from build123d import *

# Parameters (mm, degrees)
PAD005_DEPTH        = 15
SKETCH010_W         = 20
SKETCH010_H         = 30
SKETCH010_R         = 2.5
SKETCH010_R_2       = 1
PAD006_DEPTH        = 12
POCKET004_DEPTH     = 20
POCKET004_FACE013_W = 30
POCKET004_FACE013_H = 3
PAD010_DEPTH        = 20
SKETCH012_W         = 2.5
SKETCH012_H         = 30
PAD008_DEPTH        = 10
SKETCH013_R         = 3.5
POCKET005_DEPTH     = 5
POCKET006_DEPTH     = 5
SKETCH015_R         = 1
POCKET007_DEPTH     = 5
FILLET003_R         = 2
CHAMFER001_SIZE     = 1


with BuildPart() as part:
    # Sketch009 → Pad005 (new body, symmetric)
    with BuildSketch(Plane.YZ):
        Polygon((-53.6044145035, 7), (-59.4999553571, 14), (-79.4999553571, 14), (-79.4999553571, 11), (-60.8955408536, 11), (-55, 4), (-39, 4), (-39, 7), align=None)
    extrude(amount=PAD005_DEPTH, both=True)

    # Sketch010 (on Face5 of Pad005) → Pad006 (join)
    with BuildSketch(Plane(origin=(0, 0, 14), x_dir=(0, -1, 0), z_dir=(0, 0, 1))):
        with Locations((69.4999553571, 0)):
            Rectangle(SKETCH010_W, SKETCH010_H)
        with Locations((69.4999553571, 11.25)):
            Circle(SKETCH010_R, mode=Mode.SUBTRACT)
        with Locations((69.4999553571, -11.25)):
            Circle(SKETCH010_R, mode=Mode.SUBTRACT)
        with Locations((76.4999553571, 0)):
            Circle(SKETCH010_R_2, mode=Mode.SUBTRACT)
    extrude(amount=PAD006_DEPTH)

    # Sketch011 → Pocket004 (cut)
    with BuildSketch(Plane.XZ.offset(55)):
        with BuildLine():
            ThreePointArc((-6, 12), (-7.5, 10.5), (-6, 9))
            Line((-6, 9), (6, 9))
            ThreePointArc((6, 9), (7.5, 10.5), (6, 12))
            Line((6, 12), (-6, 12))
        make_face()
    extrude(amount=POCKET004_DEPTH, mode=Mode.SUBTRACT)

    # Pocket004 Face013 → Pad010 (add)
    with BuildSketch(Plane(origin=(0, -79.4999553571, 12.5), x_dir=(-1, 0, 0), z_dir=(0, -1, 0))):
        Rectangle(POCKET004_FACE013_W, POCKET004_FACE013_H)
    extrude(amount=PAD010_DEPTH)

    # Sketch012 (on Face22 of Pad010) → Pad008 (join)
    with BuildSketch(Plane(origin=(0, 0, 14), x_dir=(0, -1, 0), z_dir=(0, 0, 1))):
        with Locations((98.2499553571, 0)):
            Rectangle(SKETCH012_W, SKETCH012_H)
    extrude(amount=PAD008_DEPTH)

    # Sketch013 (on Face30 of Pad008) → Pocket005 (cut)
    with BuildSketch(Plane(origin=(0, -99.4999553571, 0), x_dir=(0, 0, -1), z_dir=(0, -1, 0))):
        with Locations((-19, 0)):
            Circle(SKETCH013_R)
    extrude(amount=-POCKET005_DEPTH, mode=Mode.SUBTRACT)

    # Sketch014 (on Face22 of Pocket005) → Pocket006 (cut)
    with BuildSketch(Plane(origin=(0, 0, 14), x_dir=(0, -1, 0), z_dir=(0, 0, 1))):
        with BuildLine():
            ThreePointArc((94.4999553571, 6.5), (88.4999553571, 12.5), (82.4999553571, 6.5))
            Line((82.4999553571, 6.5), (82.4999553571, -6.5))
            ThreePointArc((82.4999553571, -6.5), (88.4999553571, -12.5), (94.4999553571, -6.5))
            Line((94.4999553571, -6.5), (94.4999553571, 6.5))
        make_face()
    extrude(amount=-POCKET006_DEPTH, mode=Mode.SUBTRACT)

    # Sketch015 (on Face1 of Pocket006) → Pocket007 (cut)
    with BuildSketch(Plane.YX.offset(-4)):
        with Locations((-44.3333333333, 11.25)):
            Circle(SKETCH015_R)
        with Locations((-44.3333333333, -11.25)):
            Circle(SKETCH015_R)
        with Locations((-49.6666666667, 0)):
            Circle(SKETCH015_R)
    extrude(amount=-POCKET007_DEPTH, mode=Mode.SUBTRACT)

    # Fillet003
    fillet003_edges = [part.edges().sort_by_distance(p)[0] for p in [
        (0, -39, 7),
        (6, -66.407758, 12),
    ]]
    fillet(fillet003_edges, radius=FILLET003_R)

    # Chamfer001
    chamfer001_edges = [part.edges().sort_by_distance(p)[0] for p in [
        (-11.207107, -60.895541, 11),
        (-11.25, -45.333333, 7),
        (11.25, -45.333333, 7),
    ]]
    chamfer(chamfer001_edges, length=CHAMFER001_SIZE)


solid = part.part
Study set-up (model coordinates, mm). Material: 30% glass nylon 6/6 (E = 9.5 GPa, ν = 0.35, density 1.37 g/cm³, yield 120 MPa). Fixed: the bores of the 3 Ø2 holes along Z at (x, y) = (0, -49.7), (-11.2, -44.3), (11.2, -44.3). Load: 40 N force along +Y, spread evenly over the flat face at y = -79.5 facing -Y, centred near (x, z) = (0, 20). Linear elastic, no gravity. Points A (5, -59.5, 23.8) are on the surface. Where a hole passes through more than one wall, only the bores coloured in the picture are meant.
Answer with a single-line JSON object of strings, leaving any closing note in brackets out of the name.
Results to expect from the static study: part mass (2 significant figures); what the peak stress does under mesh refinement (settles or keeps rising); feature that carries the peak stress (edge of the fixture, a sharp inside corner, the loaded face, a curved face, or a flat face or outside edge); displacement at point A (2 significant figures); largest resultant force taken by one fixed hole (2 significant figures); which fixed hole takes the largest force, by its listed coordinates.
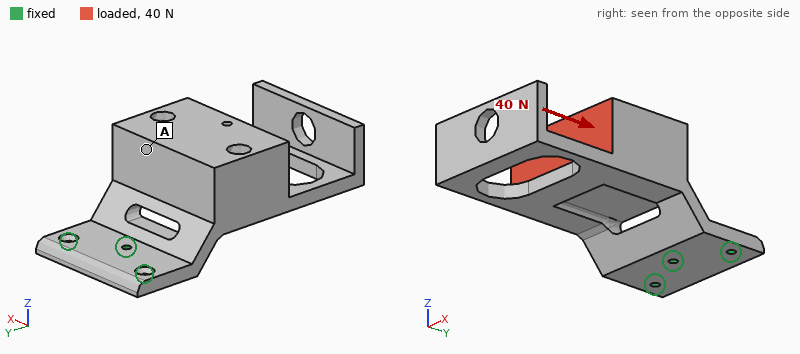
{"part mass": "16 g", "what the peak stress does under mesh refinement": "keeps rising", "feature that carries the peak stress": "edge of the fixture", "displacement at point A": "0.27 mm", "largest resultant force taken by one fixed hole": "47 N", "which fixed hole takes the largest force, by its listed coordinates": "(0, -49.7)"}
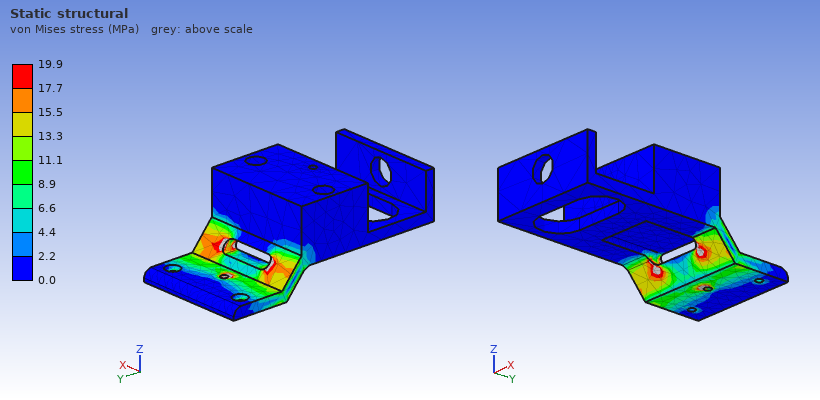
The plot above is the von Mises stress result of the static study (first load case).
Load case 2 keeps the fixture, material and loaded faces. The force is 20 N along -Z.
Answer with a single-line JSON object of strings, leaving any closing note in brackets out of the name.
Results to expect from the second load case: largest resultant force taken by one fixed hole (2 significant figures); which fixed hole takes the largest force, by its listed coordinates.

{"largest resultant force taken by one fixed hole": "59 N", "which fixed hole takes the largest force, by its listed coordinates": "(0, -49.7)"}
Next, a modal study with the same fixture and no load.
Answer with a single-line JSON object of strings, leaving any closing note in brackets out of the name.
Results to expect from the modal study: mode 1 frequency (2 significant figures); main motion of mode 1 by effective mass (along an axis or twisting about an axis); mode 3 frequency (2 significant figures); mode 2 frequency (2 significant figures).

{"mode 1 frequency": "300 Hz", "main motion of mode 1 by effective mass": "along Z", "mode 3 frequency": "1300 Hz", "mode 2 frequency": "1200 Hz"}
